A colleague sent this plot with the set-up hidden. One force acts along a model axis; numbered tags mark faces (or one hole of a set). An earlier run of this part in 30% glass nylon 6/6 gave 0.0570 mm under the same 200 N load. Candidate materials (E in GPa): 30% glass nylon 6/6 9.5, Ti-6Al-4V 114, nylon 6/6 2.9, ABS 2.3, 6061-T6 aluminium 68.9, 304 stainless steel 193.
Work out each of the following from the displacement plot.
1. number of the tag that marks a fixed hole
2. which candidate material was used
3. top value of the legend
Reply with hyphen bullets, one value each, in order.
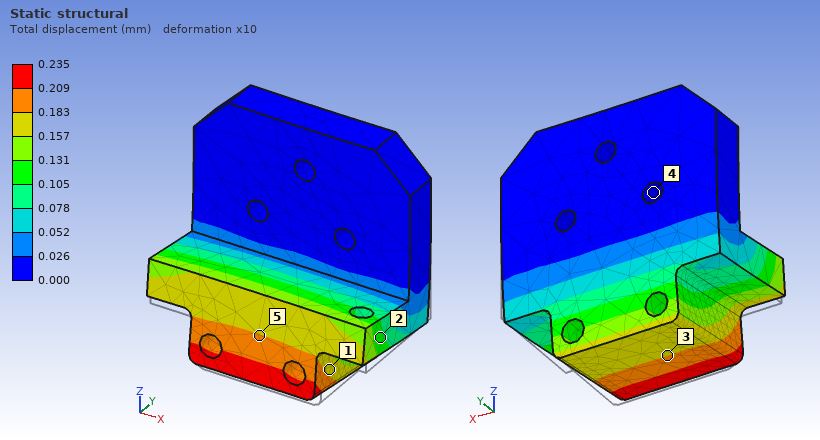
- 4
- ABS
- 0.235 mm
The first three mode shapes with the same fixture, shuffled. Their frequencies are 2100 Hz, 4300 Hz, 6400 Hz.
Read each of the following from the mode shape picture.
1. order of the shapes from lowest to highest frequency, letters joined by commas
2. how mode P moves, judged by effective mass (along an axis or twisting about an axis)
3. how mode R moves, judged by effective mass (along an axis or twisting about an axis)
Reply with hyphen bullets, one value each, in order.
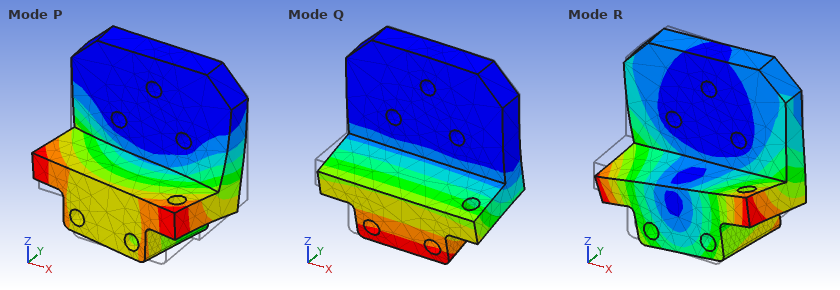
- Q, P, R
- along X
- along X
